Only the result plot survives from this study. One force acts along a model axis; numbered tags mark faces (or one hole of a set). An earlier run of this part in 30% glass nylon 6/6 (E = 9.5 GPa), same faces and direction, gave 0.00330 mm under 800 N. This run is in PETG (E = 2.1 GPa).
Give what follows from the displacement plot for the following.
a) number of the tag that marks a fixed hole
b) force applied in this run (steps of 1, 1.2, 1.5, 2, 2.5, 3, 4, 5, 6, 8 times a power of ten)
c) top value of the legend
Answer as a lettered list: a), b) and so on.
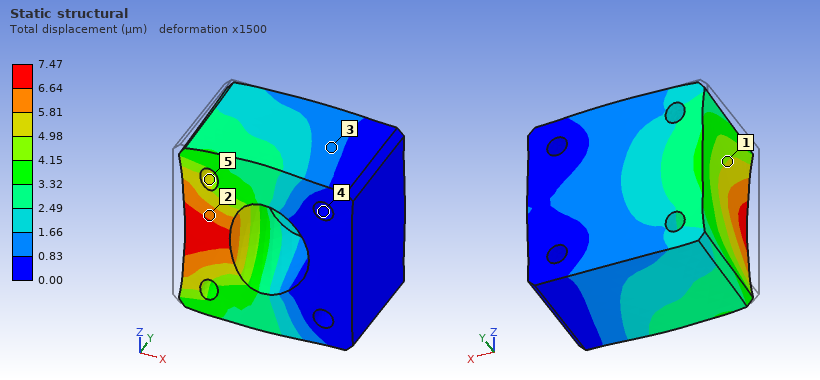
a) 4
b) 400 N
c) 7.47 µm
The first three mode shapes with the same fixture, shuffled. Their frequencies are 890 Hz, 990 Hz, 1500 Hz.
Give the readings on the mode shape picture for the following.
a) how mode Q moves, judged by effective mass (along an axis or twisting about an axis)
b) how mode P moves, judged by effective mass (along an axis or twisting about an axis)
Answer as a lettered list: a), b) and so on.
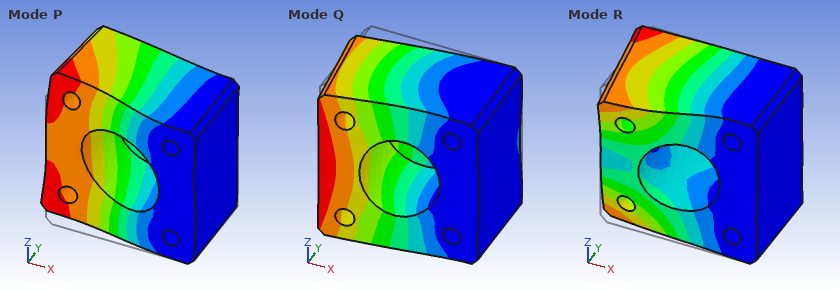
a) along Y
b) along Z
